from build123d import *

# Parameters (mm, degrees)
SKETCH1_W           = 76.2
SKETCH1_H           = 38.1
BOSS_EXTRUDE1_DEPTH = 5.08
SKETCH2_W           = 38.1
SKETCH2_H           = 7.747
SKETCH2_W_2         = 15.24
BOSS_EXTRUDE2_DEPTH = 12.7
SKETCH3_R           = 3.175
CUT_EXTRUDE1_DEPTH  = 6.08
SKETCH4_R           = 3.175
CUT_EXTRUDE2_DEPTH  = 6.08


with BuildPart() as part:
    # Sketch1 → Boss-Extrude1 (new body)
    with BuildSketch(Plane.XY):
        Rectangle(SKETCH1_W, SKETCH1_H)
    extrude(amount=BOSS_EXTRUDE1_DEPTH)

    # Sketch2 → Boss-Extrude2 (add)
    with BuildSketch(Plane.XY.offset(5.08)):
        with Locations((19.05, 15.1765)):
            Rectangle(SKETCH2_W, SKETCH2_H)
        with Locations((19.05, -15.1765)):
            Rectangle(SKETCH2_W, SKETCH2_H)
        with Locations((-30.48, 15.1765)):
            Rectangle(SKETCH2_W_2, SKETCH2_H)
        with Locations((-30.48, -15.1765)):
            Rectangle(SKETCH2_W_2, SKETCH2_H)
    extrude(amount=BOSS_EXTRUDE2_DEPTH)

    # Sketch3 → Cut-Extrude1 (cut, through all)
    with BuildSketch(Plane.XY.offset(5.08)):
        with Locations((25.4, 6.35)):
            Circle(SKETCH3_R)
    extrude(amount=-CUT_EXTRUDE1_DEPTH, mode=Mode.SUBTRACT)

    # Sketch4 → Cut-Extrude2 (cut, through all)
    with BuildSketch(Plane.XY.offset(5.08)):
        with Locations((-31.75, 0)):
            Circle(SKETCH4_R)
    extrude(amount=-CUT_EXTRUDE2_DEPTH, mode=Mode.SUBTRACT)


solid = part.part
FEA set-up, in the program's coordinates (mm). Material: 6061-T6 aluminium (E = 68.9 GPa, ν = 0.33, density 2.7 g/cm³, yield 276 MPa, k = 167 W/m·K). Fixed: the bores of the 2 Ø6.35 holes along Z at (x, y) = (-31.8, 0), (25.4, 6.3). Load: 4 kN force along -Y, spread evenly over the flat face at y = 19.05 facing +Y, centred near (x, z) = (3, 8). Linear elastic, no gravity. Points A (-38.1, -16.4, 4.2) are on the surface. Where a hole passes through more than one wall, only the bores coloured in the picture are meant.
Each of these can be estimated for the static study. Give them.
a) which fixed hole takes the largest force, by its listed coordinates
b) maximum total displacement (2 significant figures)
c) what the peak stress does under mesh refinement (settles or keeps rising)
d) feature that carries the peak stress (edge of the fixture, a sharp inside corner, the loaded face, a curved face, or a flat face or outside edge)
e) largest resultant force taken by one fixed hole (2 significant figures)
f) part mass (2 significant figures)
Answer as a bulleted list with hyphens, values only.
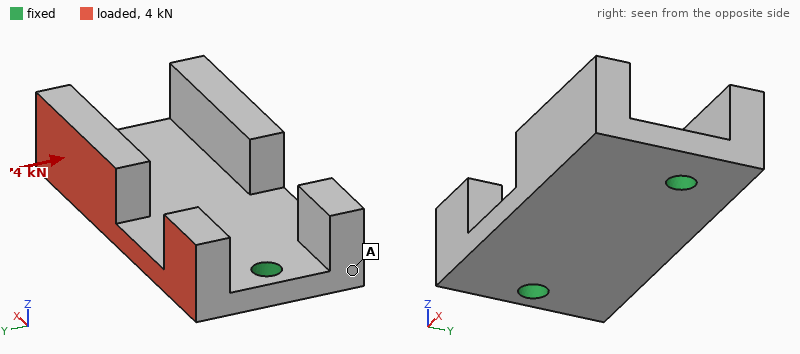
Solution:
- (25.4, 6.3)
- 0.10 mm
- keeps rising
- edge of the fixture
- 2.4 kN
- 67 g
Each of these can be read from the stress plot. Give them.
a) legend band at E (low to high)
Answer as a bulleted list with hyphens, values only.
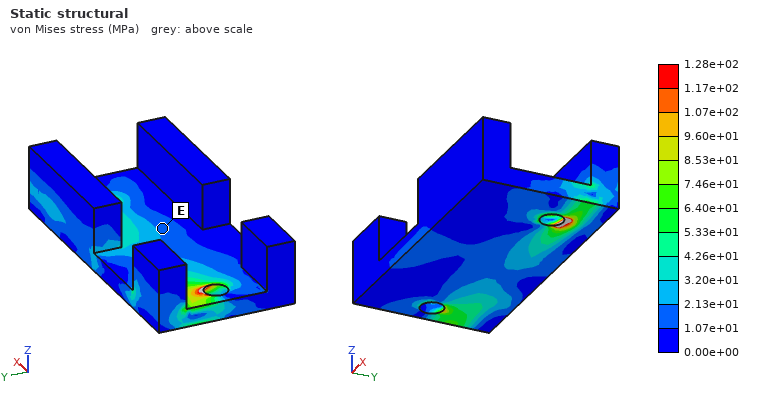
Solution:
- 1.07e+01 to 2.13e+01 MPa
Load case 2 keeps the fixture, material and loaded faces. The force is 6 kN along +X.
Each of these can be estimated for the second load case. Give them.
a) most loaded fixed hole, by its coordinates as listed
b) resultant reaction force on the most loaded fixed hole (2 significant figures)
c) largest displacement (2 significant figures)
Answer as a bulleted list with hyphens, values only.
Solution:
- (25.4, 6.3)
- 4.2 kN
- 56 µm
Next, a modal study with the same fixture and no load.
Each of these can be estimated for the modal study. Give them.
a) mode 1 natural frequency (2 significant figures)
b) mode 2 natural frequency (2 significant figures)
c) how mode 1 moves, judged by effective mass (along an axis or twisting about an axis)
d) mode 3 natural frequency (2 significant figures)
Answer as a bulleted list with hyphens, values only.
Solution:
- 3500 Hz
- 5800 Hz
- along Z
- 6000 Hz
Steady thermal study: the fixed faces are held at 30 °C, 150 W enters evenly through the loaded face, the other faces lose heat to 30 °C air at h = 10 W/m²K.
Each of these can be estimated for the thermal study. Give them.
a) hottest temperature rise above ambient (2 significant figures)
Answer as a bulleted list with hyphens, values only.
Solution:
- 49 K
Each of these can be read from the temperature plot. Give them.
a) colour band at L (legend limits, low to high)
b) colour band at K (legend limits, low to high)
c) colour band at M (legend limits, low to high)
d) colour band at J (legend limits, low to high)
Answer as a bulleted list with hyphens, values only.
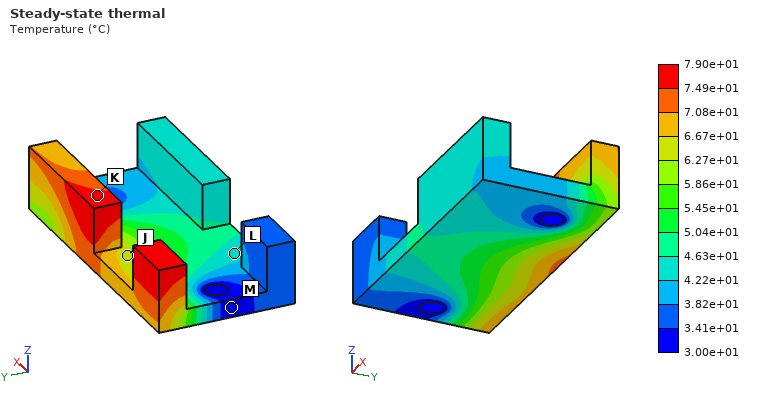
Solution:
- 4.22e+01 to 4.63e+01 °C
- 7.49e+01 to 7.90e+01 °C
- 3.00e+01 to 3.41e+01 °C
- 6.27e+01 to 6.67e+01 °C
